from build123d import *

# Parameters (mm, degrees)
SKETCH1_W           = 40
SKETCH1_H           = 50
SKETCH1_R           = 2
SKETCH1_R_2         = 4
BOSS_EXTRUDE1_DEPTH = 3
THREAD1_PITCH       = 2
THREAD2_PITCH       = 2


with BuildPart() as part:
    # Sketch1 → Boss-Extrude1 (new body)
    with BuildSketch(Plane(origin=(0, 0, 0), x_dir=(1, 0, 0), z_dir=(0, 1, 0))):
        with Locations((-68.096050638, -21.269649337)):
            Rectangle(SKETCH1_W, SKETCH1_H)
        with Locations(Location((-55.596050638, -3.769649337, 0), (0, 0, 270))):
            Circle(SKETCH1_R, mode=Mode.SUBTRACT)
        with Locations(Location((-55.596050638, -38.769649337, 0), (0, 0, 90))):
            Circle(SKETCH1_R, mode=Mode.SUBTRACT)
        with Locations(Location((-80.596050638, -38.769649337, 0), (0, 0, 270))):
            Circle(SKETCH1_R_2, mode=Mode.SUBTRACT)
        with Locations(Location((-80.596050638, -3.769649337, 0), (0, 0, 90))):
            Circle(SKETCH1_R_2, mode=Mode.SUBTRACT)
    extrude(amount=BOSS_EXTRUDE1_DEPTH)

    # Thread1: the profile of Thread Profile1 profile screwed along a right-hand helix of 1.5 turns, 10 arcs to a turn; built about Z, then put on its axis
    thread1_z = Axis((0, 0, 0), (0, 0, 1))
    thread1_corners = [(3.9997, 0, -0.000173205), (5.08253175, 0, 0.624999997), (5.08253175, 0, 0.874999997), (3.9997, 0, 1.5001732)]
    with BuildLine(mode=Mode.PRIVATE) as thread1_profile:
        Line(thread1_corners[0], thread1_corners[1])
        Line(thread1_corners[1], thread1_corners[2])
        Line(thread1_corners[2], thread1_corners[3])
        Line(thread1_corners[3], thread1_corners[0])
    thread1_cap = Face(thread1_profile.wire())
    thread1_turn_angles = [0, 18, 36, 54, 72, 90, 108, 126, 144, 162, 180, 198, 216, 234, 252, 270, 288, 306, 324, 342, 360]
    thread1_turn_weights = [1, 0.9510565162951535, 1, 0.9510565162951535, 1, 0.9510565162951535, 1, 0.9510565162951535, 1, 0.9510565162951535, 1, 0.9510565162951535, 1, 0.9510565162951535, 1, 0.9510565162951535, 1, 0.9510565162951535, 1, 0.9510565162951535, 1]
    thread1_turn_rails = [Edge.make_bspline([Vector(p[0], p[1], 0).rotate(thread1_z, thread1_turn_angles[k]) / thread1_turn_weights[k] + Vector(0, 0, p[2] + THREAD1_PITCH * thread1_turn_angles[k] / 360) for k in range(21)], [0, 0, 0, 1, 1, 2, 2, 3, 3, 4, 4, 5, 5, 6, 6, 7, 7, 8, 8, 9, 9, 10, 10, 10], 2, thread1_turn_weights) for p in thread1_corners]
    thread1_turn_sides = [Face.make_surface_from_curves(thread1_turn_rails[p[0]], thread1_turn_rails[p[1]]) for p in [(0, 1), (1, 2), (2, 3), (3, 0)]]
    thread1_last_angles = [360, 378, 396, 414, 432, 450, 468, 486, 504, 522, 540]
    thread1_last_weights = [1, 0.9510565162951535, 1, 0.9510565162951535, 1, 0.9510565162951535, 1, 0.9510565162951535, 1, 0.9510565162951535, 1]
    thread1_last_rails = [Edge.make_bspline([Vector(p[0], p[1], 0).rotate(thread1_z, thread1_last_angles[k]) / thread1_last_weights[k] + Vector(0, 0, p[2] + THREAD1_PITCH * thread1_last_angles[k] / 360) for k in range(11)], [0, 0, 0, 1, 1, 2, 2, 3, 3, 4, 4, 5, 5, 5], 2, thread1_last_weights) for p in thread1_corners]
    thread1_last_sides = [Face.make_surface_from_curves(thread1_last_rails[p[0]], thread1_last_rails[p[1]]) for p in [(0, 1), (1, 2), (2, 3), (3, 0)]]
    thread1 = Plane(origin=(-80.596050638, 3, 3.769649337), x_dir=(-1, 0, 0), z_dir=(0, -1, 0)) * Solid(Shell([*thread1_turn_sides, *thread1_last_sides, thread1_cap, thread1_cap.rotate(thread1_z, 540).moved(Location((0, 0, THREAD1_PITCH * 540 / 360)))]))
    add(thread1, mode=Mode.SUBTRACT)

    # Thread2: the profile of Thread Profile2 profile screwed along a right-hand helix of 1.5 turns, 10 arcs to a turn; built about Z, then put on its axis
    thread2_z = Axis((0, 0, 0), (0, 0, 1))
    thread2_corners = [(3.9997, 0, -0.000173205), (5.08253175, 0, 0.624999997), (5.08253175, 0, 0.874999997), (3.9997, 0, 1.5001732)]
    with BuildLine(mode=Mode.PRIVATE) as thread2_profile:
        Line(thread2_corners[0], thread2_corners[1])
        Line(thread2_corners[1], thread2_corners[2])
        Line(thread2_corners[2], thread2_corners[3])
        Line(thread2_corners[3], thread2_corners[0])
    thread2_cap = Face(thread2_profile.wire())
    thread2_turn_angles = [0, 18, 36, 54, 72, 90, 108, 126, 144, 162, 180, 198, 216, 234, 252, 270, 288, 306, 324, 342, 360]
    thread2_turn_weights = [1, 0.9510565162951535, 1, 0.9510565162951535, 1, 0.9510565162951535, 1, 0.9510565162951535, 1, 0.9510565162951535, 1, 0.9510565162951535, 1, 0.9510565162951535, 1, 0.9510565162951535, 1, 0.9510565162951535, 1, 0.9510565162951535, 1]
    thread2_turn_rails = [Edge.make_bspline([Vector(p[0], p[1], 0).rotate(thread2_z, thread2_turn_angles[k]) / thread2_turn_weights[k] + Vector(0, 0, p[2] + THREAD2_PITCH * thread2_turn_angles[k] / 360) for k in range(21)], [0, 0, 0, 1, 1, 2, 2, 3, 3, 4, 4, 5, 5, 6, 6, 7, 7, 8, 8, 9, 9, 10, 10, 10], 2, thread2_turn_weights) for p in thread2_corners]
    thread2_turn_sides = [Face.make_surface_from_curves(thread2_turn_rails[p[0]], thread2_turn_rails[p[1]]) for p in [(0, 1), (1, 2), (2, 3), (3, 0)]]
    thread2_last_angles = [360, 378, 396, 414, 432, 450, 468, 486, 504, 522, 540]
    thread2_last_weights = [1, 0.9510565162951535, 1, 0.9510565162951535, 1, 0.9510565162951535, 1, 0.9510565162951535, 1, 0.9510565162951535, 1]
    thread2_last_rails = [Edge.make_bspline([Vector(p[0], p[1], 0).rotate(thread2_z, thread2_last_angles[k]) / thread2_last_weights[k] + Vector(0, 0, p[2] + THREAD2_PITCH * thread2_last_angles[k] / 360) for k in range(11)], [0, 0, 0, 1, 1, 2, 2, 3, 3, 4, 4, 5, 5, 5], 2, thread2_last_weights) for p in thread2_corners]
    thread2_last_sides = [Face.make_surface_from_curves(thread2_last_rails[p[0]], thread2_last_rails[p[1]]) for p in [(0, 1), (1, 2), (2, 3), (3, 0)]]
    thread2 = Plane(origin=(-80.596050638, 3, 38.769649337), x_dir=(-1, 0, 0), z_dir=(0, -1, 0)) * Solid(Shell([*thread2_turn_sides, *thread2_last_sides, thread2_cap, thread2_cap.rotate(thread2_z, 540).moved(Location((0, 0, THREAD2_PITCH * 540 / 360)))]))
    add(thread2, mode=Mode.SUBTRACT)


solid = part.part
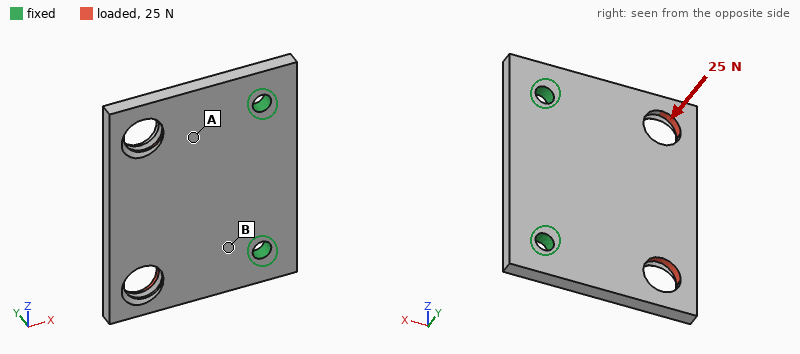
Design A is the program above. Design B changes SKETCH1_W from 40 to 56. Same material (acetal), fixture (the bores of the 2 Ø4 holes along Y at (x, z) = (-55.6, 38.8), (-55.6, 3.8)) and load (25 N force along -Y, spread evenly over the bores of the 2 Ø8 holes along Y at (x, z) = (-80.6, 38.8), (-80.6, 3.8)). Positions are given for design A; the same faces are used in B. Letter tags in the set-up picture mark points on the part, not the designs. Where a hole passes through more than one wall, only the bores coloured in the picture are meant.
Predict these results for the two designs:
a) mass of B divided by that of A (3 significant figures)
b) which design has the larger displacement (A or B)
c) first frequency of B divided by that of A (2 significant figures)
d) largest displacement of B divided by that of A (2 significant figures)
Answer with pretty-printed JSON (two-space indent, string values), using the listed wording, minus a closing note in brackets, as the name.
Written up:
{
  "mass of B divided by that of A": "1.43",
  "which design has the larger displacement": "B",
  "first frequency of B divided by that of A": "0.63",
  "largest displacement of B divided by that of A": "1.3"
}
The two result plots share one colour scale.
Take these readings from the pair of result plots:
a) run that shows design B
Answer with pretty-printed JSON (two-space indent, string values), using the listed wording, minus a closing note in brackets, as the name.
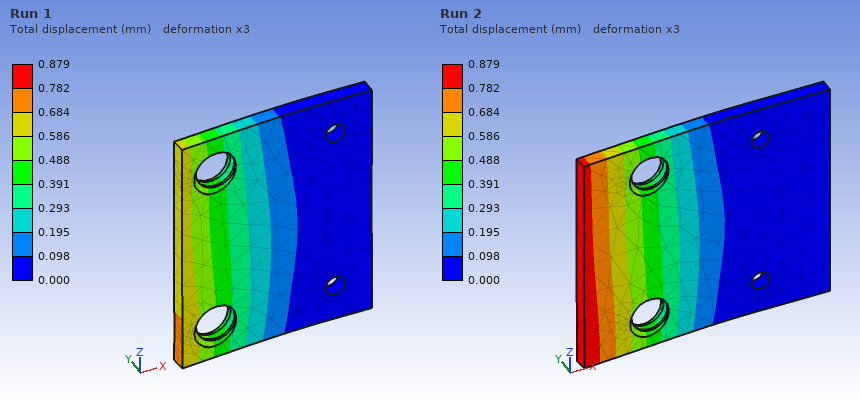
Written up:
{
  "run that shows design B": "Run 2"
}
